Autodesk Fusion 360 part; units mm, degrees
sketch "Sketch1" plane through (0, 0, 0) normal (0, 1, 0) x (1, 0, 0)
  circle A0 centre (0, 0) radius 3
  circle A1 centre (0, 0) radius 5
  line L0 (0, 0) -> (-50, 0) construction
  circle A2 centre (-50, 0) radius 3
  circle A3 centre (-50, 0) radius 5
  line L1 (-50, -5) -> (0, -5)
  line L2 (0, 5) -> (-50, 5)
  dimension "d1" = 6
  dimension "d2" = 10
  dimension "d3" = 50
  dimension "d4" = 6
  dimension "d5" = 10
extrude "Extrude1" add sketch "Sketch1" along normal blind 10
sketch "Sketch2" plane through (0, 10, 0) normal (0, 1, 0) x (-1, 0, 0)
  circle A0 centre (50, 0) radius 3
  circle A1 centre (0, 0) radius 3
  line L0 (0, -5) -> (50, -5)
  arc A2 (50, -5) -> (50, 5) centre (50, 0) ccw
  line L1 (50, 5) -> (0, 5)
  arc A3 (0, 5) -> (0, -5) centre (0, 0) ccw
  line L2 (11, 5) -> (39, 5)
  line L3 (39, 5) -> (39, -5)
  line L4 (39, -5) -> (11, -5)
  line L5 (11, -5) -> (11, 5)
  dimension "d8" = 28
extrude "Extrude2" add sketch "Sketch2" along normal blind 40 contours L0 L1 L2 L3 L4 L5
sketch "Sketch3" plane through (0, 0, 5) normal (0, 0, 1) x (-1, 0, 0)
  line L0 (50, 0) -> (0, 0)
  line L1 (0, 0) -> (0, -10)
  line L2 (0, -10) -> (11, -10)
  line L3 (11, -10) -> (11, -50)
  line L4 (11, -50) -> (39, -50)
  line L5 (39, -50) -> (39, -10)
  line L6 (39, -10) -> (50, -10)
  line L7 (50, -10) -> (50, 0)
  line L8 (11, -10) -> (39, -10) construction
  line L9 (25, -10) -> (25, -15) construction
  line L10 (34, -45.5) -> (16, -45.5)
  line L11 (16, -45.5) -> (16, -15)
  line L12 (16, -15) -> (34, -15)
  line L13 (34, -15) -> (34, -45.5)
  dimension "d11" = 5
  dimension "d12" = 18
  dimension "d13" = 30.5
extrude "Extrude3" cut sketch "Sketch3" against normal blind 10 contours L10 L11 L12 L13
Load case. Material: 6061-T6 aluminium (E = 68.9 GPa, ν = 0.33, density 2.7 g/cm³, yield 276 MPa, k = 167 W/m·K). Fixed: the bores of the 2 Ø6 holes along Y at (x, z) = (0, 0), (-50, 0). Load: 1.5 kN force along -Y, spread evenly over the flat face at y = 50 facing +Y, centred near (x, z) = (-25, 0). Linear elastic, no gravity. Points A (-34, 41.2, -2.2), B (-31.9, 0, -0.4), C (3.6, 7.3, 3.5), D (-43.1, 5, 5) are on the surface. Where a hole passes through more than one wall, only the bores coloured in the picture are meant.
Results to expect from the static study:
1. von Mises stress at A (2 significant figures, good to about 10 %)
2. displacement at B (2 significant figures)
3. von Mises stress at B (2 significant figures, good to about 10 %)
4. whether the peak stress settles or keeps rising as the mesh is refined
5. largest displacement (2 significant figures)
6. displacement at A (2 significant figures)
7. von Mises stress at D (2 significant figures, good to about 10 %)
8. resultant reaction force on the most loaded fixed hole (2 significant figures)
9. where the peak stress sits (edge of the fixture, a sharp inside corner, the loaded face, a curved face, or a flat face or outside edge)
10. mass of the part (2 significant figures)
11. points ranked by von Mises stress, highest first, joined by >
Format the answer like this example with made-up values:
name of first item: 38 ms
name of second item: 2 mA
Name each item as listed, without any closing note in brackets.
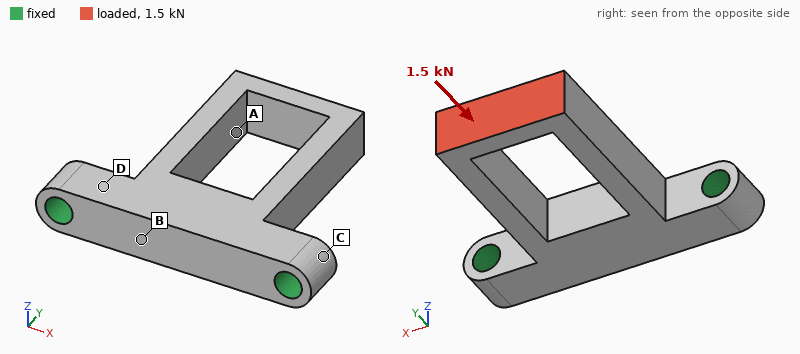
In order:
von Mises stress at A: 42 MPa
displacement at B: 6.4 µm
von Mises stress at B: 9.2 MPa
whether the peak stress settles or keeps rising as the mesh is refined: keeps rising
largest displacement: 32 µm
displacement at A: 17 µm
von Mises stress at D: 20 MPa
resultant reaction force on the most loaded fixed hole: 770 N
where the peak stress sits: edge of the fixture
mass of the part: 30 g
points ranked by von Mises stress, highest first, joined by >: A > D > B > C
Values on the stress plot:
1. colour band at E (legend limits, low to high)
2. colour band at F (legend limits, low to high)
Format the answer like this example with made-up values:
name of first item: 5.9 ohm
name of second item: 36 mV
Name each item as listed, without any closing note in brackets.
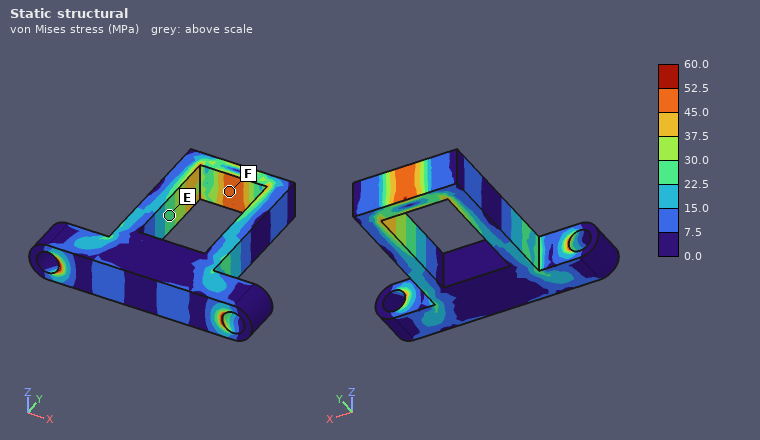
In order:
colour band at E: 22.5 to 30.0 MPa
colour band at F: 45.0 to 52.5 MPa
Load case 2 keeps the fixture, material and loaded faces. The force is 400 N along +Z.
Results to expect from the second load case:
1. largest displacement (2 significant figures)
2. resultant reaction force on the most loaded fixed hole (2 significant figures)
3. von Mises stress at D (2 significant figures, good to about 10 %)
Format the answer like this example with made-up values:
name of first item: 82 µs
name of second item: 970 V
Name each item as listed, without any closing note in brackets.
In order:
largest displacement: 0.29 mm
resultant reaction force on the most loaded fixed hole: 200 N
von Mises stress at D: 76 MPa
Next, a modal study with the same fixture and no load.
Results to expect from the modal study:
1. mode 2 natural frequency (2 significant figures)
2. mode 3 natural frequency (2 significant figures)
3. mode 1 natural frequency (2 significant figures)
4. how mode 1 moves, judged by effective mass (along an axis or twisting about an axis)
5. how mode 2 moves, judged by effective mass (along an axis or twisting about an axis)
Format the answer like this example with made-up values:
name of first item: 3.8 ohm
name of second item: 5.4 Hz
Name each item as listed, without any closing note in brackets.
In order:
mode 2 natural frequency: 3400 Hz
mode 3 natural frequency: 6200 Hz
mode 1 natural frequency: 2600 Hz
how mode 1 moves, judged by effective mass: along Z
how mode 2 moves, judged by effective mass: along X
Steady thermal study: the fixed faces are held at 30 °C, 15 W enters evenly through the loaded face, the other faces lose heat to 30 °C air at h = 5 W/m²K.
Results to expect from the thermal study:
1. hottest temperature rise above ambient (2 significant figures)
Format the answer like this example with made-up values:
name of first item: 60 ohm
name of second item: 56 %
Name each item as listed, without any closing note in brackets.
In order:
hottest temperature rise above ambient: 42 K
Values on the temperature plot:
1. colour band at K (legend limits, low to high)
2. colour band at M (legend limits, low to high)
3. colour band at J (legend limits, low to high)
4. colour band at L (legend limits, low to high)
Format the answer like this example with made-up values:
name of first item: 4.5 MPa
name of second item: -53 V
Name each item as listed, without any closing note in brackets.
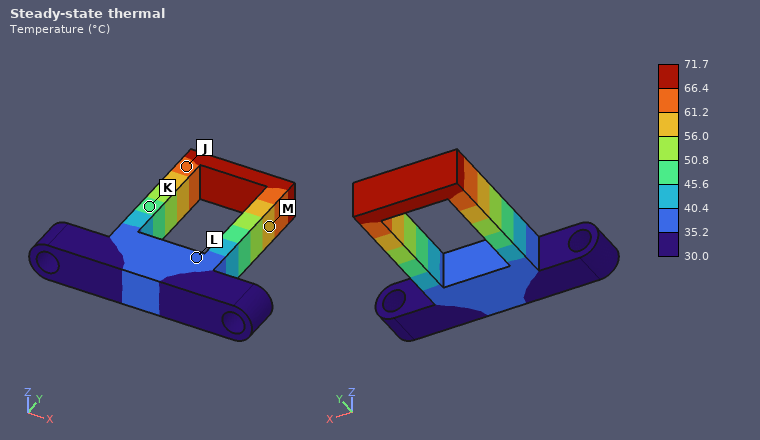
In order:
colour band at K: 45.6 to 50.8 °C
colour band at M: 56.0 to 61.2 °C
colour band at J: 61.2 to 66.4 °C
colour band at L: 35.2 to 40.4 °C
